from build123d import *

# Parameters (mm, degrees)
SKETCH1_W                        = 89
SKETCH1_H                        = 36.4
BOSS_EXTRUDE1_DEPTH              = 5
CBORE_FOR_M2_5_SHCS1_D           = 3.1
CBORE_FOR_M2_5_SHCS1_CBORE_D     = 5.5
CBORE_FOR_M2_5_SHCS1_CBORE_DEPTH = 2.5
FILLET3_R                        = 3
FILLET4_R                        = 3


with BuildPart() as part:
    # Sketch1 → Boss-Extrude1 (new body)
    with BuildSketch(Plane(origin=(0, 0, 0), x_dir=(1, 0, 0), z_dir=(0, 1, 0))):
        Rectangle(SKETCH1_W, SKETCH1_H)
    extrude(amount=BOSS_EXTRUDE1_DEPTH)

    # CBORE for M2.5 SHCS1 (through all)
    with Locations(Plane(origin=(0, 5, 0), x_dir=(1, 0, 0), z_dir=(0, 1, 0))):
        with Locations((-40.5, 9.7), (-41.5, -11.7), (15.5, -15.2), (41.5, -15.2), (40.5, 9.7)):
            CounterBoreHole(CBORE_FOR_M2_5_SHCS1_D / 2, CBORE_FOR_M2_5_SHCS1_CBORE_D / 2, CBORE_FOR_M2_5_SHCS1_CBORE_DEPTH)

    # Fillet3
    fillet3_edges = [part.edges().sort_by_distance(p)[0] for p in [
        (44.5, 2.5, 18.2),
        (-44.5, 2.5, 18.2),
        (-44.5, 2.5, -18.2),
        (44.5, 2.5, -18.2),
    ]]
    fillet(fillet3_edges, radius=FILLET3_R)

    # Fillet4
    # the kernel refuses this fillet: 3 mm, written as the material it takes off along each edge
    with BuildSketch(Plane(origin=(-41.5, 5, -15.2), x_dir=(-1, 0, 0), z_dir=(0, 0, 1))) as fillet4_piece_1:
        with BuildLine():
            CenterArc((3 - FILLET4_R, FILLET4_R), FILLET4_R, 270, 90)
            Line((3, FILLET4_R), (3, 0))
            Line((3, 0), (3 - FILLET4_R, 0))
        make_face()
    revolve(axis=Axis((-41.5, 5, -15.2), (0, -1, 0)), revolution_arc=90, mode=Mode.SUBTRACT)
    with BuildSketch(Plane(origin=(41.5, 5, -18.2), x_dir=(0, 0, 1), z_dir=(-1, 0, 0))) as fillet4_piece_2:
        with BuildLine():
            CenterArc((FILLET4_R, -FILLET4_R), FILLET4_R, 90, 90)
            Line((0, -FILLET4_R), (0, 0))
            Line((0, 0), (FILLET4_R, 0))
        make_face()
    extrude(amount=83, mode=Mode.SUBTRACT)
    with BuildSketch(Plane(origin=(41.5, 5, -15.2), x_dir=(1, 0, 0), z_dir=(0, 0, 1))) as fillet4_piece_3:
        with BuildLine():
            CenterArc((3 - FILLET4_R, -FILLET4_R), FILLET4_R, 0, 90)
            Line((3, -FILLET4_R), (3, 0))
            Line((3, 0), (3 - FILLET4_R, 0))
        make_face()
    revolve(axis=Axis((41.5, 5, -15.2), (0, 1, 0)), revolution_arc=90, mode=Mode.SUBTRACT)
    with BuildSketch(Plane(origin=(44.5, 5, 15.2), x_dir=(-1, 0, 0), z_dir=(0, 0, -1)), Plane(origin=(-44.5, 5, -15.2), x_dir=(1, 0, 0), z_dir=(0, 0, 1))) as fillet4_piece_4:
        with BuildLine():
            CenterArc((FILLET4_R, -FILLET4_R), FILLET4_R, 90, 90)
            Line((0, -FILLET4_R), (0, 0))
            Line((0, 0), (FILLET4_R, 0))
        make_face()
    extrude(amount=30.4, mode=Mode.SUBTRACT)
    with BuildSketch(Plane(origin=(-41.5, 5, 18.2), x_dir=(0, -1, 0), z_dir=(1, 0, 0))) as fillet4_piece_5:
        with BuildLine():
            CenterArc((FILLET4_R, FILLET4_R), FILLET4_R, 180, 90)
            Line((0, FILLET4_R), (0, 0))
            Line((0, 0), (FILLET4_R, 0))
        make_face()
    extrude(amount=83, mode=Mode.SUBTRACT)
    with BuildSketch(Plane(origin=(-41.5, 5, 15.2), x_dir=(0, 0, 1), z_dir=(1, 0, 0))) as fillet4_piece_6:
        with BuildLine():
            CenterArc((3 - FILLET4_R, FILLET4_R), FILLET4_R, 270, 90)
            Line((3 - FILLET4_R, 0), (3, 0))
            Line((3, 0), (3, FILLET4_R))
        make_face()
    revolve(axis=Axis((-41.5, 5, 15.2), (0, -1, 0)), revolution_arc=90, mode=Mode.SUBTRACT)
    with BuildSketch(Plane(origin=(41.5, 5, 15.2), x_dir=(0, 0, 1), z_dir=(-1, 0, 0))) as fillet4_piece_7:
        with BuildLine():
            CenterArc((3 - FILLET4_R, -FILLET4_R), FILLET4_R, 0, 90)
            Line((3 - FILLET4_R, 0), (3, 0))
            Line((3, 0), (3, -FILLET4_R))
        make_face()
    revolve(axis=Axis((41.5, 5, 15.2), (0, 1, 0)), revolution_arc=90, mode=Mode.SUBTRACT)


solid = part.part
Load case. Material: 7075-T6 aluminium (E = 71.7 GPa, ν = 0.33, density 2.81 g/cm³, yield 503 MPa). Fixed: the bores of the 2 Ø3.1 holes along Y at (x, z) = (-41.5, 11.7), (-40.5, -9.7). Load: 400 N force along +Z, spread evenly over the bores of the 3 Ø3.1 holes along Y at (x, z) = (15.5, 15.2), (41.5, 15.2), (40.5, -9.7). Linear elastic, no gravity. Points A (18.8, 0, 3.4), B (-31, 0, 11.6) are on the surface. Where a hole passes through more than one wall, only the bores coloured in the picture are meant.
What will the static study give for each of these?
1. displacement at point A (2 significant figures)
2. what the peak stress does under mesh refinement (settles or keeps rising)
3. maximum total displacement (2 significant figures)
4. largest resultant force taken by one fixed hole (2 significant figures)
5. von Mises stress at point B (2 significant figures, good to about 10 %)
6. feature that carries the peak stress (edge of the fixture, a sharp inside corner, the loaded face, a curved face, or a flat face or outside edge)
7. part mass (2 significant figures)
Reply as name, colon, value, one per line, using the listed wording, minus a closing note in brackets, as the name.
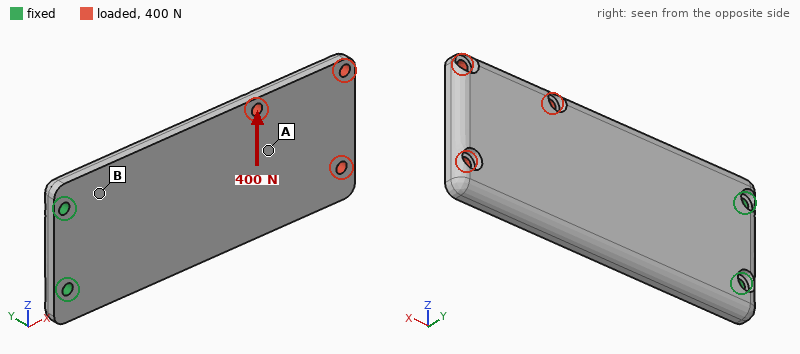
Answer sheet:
displacement at point A: 56 µm
what the peak stress does under mesh refinement: keeps rising
maximum total displacement: 94 µm
largest resultant force taken by one fixed hole: 1.3 kN
von Mises stress at point B: 27 MPa
feature that carries the peak stress: edge of the fixture
part mass: 43 g
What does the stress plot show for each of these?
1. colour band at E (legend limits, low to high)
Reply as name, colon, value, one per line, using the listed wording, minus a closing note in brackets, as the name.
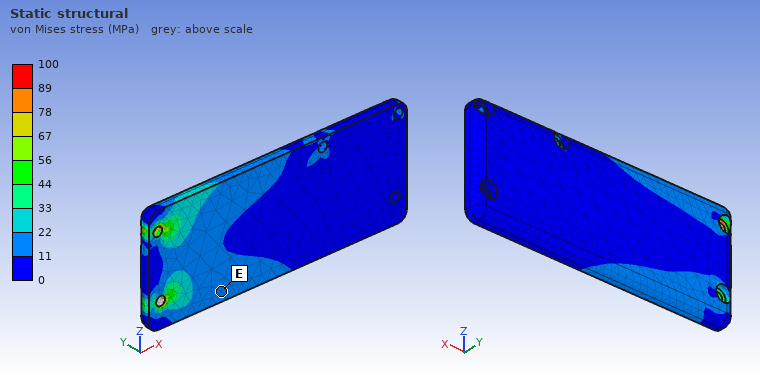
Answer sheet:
colour band at E: 11 to 22 MPa
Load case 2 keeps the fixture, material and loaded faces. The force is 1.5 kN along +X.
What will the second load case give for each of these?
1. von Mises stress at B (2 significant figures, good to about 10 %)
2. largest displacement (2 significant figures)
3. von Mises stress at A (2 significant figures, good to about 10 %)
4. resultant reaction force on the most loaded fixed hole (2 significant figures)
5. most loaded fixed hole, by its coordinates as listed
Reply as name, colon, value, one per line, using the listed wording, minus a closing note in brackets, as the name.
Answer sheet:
von Mises stress at B: 32 MPa
largest displacement: 0.24 mm
von Mises stress at A: 17 MPa
resultant reaction force on the most loaded fixed hole: 1.1 kN
most loaded fixed hole, by its coordinates as listed: (-41.5, 11.7)
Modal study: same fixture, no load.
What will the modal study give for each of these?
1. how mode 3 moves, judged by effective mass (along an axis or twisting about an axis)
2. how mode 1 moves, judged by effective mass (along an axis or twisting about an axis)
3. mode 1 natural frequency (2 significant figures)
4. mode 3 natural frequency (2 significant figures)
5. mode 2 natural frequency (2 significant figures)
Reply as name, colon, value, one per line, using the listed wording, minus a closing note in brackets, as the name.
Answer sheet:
how mode 3 moves, judged by effective mass: along Z
how mode 1 moves, judged by effective mass: along Y
mode 1 natural frequency: 460 Hz
mode 3 natural frequency: 3000 Hz
mode 2 natural frequency: 2500 Hz
